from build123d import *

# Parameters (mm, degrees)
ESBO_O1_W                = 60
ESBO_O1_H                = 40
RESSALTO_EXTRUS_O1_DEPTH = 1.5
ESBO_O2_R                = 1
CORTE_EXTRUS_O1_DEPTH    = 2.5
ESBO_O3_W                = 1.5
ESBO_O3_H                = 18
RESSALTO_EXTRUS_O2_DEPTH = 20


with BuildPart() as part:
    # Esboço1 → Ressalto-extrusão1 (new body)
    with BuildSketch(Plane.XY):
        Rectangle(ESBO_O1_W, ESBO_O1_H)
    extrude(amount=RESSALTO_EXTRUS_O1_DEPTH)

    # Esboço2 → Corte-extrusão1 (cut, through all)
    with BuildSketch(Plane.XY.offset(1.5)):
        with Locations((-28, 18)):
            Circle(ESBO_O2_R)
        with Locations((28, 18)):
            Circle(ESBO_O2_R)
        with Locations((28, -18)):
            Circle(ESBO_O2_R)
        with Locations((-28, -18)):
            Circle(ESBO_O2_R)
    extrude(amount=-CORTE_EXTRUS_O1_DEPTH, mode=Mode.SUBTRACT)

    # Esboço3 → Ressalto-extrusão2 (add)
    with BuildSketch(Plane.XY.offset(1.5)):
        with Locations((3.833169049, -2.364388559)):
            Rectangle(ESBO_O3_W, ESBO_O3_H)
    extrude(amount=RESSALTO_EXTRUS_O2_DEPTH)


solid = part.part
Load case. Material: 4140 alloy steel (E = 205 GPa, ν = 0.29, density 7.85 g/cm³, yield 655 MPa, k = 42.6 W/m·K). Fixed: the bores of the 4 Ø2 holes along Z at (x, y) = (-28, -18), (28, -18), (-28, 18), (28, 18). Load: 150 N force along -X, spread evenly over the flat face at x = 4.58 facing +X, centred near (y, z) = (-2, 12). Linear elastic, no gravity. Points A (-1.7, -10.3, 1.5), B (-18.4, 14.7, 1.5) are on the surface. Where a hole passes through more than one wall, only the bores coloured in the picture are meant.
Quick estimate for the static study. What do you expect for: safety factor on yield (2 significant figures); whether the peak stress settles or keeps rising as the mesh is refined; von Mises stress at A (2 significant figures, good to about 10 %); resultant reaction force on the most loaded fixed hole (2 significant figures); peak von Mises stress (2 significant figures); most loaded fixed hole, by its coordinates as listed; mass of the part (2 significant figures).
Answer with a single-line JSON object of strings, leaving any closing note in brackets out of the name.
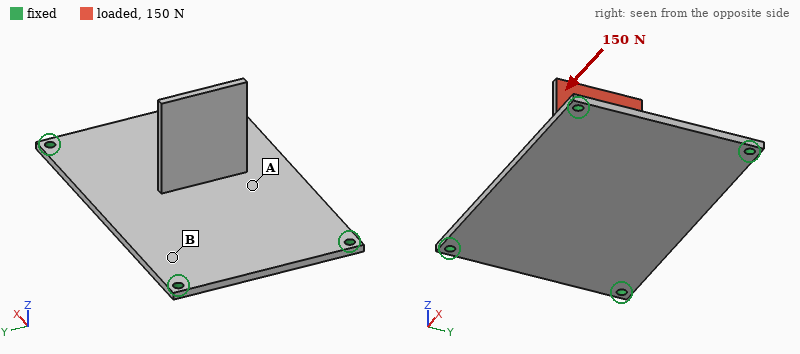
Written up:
{"safety factor on yield": "2.9", "whether the peak stress settles or keeps rising as the mesh is refined": "settles", "von Mises stress at A": "47 MPa", "resultant reaction force on the most loaded fixed hole": "50 N", "peak von Mises stress": "220 MPa", "most loaded fixed hole, by its coordinates as listed": "(28, -18)", "mass of the part": "32 g"}
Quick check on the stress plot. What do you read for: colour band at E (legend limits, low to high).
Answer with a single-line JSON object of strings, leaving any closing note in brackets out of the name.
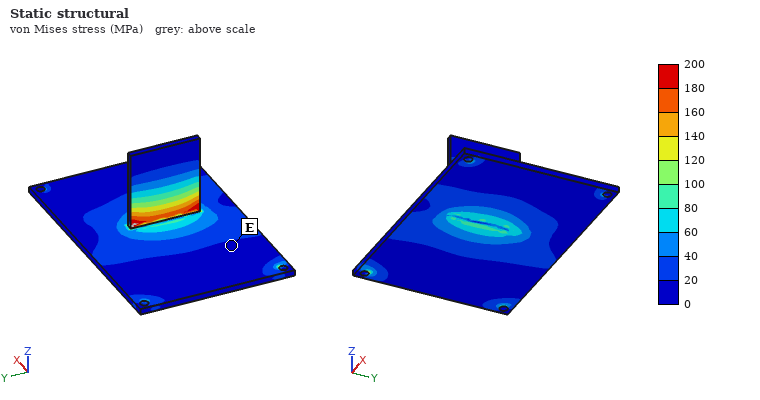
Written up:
{"colour band at E": "0 to 20 MPa"}
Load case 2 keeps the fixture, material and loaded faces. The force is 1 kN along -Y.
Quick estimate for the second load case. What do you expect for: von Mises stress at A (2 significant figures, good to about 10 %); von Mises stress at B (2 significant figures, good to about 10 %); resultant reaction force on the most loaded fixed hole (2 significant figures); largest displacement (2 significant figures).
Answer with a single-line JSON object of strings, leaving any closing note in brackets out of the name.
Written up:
{"von Mises stress at A": "190 MPa", "von Mises stress at B": "140 MPa", "resultant reaction force on the most loaded fixed hole": "400 N", "largest displacement": "0.50 mm"}
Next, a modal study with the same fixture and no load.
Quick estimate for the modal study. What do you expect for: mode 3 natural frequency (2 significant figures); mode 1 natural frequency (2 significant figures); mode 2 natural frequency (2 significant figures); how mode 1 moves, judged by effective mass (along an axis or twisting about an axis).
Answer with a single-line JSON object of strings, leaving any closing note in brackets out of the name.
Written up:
{"mode 3 natural frequency": "2700 Hz", "mode 1 natural frequency": "1700 Hz", "mode 2 natural frequency": "2500 Hz", "how mode 1 moves, judged by effective mass": "along Z"}
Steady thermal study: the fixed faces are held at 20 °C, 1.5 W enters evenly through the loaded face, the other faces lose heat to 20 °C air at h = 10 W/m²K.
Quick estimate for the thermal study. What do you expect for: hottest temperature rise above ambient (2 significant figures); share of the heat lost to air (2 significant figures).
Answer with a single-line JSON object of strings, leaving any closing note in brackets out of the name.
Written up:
{"hottest temperature rise above ambient": "23 K", "share of the heat lost to air": "24 %"}
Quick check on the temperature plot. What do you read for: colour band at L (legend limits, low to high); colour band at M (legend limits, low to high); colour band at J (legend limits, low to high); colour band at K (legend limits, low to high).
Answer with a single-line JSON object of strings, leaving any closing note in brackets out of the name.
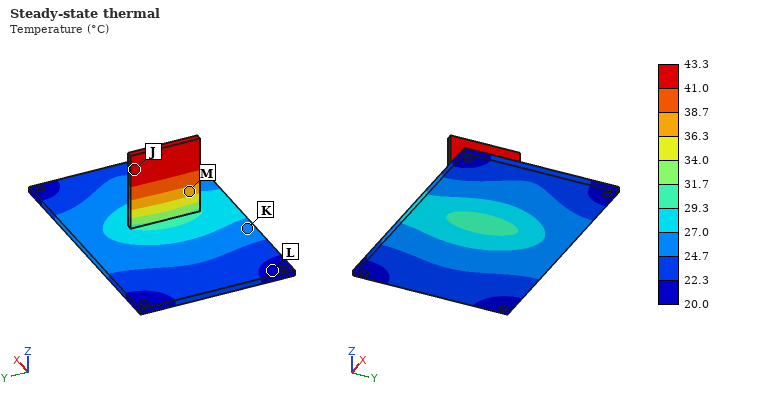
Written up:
{"colour band at L": "20.0 to 22.3 °C", "colour band at M": "36.3 to 38.7 °C", "colour band at J": "41.0 to 43.3 °C", "colour band at K": "24.7 to 27.0 °C"}
